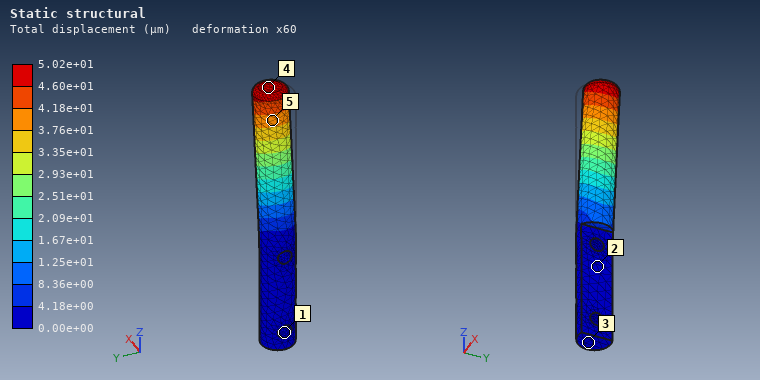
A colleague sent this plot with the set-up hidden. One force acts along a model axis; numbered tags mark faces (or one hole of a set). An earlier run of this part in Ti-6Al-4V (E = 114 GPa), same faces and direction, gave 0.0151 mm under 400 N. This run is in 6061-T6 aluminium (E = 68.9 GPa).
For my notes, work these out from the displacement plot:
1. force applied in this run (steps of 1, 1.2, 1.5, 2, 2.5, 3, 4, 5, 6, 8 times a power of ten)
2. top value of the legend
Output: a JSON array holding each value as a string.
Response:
["800 N", "5.02e+01 µm"]
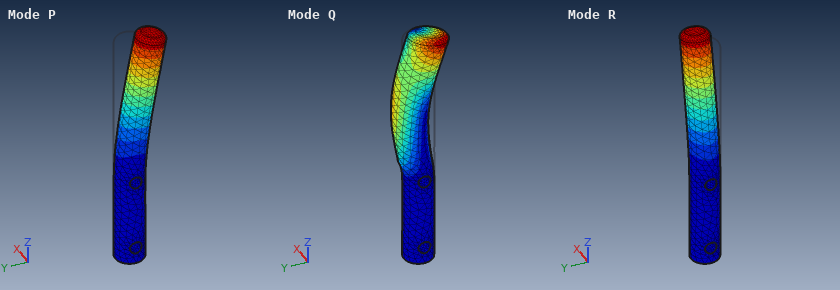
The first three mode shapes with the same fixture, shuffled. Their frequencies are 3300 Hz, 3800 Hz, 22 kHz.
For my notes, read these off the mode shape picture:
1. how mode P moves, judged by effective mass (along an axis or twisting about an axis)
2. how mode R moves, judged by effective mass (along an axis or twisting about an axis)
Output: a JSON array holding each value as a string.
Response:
["along Y", "along X"]
